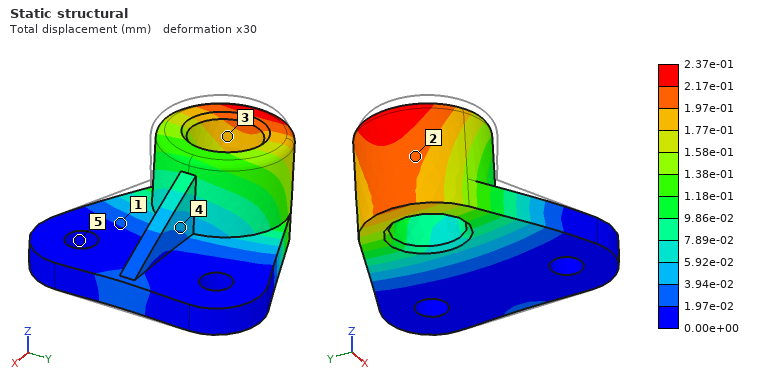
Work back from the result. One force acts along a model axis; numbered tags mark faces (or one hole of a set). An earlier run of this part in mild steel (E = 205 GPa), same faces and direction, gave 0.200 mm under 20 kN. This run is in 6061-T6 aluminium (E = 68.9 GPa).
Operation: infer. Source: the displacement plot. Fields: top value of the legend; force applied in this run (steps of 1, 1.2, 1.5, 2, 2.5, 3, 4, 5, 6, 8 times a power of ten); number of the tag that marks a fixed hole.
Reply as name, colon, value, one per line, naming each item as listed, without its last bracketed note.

top value of the legend: 2.37e-01 mm
force applied in this run: 8 kN
number of the tag that marks a fixed hole: 5
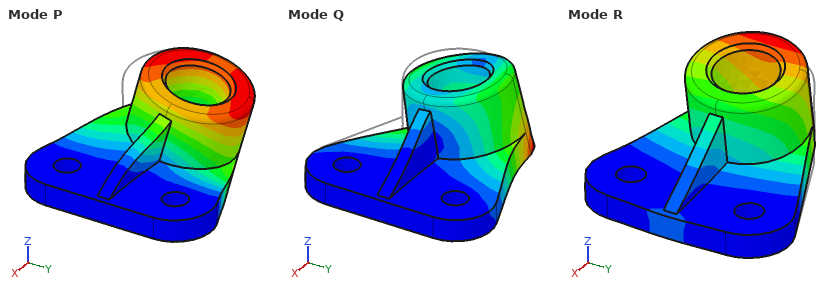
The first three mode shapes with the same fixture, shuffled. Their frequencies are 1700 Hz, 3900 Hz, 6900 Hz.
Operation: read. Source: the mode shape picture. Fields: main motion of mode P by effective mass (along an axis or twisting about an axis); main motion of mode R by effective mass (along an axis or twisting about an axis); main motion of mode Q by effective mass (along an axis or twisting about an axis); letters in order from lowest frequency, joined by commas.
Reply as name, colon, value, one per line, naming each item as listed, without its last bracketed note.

main motion of mode P by effective mass: along Y
main motion of mode R by effective mass: along Z
main motion of mode Q by effective mass: along Y
letters in order from lowest frequency, joined by commas: R, P, Q
